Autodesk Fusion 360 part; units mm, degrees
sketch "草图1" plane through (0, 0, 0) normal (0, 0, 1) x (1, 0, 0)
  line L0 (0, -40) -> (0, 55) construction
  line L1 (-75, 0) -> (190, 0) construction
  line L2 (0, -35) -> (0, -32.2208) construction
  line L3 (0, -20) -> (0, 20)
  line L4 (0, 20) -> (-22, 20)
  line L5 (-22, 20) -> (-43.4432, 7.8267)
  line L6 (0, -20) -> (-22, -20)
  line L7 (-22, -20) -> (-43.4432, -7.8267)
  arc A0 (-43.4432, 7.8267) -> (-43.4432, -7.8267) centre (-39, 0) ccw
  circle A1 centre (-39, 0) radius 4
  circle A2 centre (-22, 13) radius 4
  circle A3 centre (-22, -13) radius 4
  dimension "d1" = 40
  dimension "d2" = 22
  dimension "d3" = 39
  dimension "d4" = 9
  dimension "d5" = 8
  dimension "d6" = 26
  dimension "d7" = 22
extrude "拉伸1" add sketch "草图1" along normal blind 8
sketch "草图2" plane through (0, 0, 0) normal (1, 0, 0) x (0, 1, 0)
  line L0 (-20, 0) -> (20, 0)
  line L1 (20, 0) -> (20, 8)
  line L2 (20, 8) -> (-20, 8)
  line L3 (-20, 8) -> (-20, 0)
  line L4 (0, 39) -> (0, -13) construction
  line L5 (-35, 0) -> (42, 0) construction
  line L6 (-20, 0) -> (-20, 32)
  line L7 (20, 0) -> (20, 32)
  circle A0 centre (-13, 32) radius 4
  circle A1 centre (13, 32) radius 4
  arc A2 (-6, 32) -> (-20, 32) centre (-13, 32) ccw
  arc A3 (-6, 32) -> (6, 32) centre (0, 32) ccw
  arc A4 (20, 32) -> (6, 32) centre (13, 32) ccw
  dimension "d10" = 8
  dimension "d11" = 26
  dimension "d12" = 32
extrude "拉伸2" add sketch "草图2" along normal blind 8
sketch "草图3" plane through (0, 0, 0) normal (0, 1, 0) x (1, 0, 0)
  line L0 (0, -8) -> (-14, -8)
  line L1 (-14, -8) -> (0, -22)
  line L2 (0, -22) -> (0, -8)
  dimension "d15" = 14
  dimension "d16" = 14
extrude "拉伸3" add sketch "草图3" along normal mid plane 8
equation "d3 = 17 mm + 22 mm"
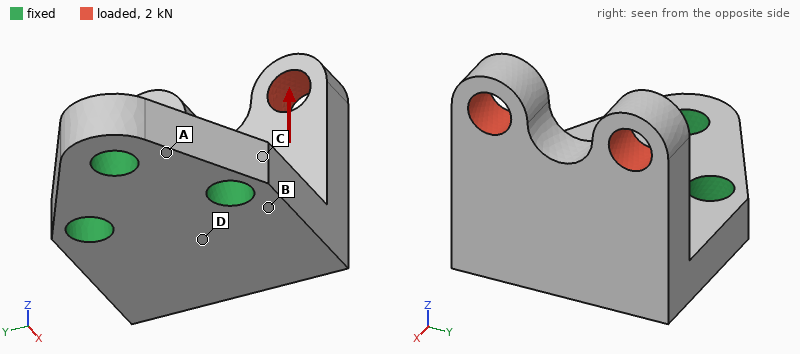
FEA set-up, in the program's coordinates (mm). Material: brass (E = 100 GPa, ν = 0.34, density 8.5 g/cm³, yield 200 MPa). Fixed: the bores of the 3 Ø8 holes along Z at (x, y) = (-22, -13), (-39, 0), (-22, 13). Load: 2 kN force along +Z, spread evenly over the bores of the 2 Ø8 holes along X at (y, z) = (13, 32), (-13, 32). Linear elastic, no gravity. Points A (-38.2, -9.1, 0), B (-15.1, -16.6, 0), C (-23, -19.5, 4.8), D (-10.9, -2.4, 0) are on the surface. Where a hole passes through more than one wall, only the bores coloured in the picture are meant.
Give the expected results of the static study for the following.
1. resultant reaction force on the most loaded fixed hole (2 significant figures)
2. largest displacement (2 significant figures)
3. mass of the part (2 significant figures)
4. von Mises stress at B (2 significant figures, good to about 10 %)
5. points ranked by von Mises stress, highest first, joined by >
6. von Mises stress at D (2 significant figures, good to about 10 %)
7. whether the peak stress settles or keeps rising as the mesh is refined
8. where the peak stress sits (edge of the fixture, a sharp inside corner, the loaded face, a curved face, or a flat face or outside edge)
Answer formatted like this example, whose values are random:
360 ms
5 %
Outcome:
1.2 kN
0.12 mm
190 g
86 MPa
B > D > C > A
51 MPa
keeps rising
edge of the fixture
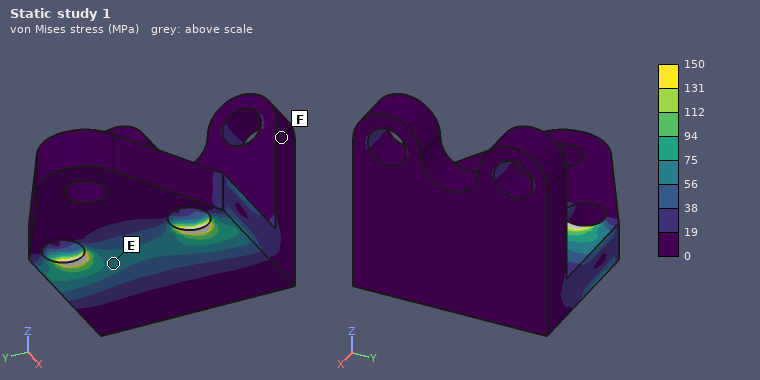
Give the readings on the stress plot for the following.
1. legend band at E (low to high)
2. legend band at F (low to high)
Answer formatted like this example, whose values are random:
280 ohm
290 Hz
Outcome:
56 to 75 MPa
0 to 19 MPa
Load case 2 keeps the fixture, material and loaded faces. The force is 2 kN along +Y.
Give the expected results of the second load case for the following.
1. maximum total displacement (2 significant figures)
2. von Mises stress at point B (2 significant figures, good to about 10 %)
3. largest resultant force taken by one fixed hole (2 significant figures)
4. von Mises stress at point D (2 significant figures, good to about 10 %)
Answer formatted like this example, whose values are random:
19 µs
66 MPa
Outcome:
0.10 mm
82 MPa
2.8 kN
41 MPa
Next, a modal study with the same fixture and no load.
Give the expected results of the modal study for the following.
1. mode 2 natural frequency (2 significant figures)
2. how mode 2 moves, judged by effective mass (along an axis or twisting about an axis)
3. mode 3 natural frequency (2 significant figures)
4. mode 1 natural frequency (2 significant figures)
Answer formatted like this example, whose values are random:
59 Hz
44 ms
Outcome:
4000 Hz
along Y
6900 Hz
2400 Hz
